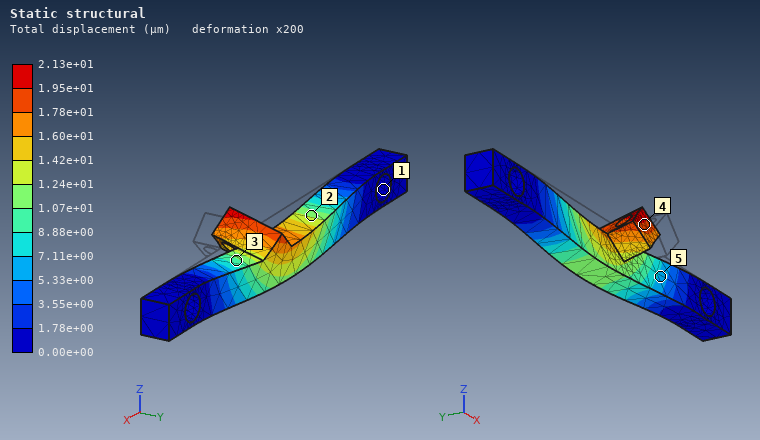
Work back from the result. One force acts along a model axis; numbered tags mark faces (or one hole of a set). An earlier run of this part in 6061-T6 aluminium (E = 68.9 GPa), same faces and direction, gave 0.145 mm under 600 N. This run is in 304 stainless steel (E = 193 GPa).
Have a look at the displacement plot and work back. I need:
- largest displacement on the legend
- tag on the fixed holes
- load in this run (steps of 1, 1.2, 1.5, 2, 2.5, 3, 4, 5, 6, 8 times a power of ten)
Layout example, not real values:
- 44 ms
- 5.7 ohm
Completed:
- 2.13e+01 µm
- 1
- 250 N
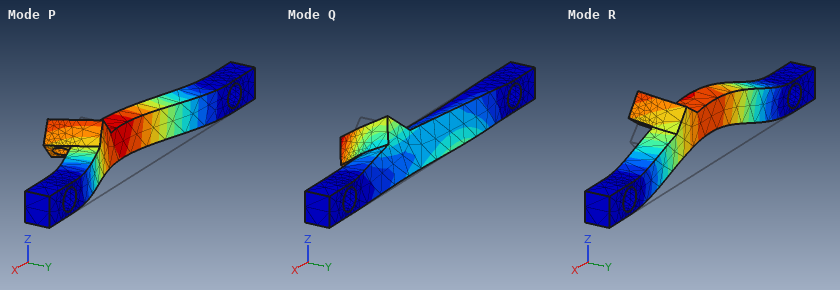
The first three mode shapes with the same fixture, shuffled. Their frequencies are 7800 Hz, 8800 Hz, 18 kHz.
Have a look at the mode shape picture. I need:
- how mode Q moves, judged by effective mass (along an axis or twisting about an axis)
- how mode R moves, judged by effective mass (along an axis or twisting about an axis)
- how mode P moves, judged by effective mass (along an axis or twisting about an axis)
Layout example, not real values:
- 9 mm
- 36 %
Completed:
- twisting about X
- along Z
- along Y
